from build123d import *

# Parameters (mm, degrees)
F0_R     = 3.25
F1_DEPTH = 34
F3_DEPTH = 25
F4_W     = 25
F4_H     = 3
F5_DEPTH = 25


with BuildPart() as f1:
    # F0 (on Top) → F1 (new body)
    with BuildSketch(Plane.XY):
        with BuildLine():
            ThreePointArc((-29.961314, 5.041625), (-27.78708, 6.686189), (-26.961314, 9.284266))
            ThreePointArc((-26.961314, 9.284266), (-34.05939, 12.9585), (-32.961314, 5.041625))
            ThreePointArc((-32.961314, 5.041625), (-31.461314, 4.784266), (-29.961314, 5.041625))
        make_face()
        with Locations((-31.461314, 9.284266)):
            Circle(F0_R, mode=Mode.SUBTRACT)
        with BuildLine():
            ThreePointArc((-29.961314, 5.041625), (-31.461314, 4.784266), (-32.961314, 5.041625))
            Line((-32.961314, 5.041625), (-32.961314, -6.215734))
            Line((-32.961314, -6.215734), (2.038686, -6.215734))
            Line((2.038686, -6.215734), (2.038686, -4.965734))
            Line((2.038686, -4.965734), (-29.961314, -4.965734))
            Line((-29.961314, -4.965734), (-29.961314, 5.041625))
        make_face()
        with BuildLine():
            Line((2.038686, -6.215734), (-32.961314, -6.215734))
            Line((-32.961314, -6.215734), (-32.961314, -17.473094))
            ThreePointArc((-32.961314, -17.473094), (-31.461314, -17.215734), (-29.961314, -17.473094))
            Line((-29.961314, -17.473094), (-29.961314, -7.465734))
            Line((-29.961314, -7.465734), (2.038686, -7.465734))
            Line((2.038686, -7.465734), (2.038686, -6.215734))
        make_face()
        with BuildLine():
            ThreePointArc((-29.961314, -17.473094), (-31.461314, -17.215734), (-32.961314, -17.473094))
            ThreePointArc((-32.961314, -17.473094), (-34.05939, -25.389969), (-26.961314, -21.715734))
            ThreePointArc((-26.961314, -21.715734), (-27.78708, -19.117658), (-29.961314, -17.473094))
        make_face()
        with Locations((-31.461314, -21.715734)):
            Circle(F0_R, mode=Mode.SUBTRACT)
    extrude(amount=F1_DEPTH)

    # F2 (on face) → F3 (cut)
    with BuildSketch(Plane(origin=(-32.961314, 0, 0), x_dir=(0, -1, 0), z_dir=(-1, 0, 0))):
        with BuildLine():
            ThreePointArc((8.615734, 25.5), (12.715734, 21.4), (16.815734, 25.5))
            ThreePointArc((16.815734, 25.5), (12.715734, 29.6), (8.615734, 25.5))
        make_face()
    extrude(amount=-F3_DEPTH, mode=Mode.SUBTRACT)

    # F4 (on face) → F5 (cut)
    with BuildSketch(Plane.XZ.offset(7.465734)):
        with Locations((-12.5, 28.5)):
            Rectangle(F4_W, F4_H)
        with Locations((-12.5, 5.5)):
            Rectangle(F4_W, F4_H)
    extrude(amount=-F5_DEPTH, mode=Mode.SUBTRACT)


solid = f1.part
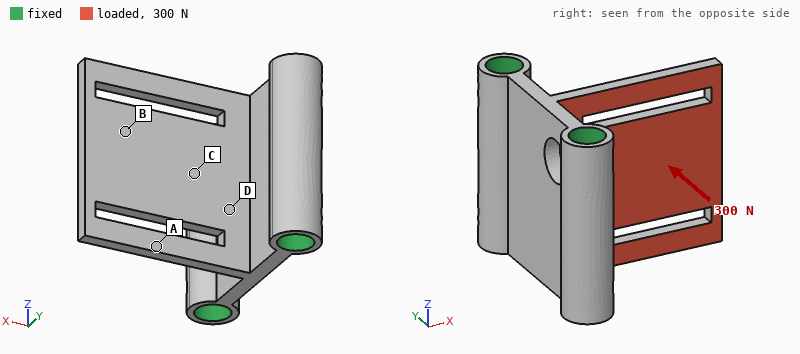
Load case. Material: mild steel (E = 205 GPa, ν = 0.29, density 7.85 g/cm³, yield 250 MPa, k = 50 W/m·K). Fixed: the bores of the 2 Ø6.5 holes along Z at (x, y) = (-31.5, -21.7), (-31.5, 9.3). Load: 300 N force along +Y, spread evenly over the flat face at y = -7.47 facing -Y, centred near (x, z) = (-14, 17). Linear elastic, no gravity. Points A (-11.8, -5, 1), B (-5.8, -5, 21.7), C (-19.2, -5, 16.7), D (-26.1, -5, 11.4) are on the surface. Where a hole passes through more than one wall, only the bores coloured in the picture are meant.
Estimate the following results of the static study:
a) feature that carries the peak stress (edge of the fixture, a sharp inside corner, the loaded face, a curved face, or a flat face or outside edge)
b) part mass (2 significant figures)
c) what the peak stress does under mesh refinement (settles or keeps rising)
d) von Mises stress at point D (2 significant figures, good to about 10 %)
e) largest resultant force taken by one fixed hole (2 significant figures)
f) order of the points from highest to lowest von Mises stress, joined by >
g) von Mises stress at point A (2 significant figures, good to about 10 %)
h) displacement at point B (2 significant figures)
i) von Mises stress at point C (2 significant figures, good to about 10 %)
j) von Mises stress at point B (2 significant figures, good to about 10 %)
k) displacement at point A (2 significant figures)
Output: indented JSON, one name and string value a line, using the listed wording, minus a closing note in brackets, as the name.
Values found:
{
  "feature that carries the peak stress": "a sharp inside corner",
  "part mass": "51 g",
  "what the peak stress does under mesh refinement": "keeps rising",
  "von Mises stress at point D": "110 MPa",
  "largest resultant force taken by one fixed hole": "360 N",
  "order of the points from highest to lowest von Mises stress, joined by >": "D > C > A > B",
  "von Mises stress at point A": "33 MPa",
  "displacement at point B": "0.12 mm",
  "von Mises stress at point C": "65 MPa",
  "von Mises stress at point B": "12 MPa",
  "displacement at point A": "0.076 mm"
}
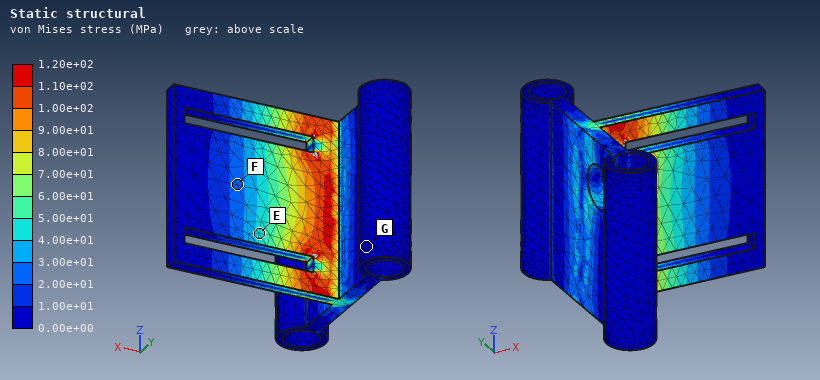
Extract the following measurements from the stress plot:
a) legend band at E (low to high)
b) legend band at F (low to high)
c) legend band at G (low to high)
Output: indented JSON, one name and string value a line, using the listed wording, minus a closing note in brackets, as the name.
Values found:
{
  "legend band at E": "4.00e+01 to 5.00e+01 MPa",
  "legend band at F": "2.00e+01 to 3.00e+01 MPa",
  "legend band at G": "0.00e+00 to 1.00e+01 MPa"
}
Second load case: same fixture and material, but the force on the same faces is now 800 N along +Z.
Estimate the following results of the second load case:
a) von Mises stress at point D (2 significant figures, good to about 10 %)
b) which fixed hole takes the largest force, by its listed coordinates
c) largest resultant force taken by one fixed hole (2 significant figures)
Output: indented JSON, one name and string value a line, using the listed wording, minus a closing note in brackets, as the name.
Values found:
{
  "von Mises stress at point D": "21 MPa",
  "which fixed hole takes the largest force, by its listed coordinates": "(-31.5, 9.3)",
  "largest resultant force taken by one fixed hole": "450 N"
}
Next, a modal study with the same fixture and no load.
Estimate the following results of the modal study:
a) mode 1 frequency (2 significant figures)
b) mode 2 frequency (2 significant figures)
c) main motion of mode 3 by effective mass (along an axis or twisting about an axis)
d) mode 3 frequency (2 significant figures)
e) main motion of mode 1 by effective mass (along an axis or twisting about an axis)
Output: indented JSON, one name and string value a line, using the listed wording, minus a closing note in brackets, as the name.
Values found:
{
  "mode 1 frequency": "1900 Hz",
  "mode 2 frequency": "4400 Hz",
  "main motion of mode 3 by effective mass": "along Z",
  "mode 3 frequency": "6600 Hz",
  "main motion of mode 1 by effective mass": "along Y"
}
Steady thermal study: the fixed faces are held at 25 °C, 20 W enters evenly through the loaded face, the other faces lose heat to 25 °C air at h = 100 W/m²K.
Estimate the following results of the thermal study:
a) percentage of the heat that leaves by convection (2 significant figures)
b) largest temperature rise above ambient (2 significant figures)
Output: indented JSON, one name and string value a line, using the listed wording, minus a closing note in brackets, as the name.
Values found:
{
  "percentage of the heat that leaves by convection": "42 %",
  "largest temperature rise above ambient": "66 K"
}
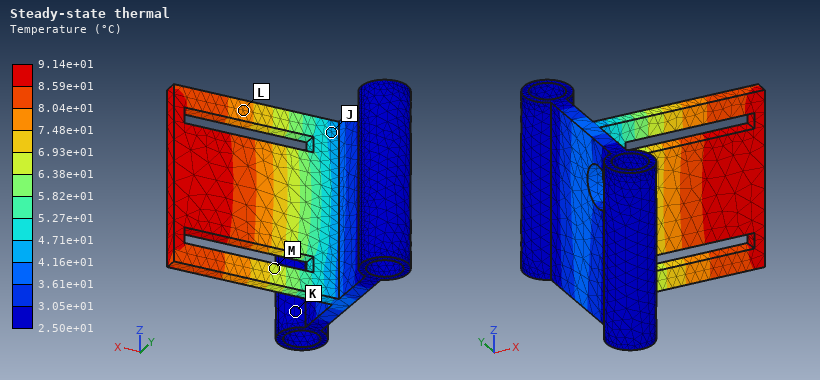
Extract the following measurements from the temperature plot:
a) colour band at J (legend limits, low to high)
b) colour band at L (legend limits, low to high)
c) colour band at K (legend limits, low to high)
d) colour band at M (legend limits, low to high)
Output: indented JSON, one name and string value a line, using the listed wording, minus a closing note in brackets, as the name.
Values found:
{
  "colour band at J": "4.16e+01 to 4.71e+01 °C",
  "colour band at L": "7.48e+01 to 8.04e+01 °C",
  "colour band at K": "2.50e+01 to 3.05e+01 °C",
  "colour band at M": "6.38e+01 to 6.93e+01 °C"
}
